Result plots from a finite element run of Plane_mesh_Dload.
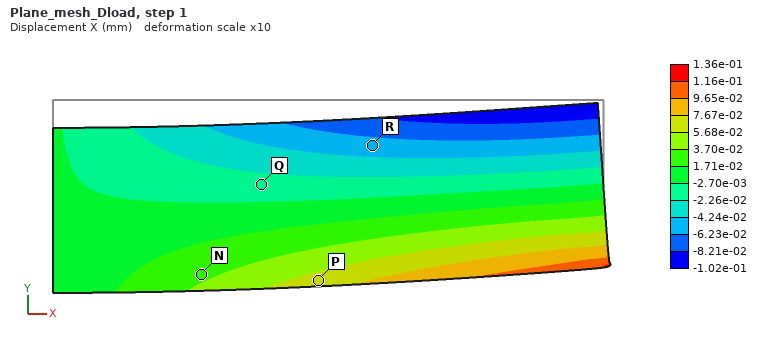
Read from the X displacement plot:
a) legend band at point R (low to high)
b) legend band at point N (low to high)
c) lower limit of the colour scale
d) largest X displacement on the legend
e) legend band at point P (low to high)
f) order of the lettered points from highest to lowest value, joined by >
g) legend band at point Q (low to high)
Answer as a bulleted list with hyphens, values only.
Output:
- -6.23e-02 to -4.24e-02 mm
- 1.71e-02 to 3.70e-02 mm
- -1.02e-01 mm
- 1.36e-01 mm
- 5.68e-02 to 7.67e-02 mm
- P > N > Q > R
- -2.26e-02 to -2.70e-03 mm
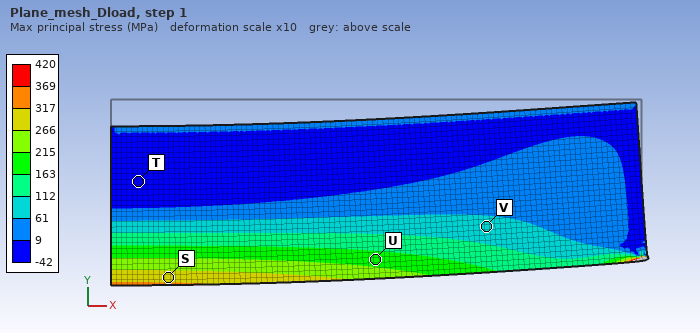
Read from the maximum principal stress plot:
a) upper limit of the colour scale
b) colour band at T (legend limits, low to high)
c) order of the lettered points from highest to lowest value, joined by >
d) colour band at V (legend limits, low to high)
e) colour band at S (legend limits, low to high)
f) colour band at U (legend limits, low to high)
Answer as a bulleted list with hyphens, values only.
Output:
- 420 MPa
- -42 to 9 MPa
- S > U > V > T
- 61 to 112 MPa
- 266 to 317 MPa
- 163 to 215 MPa
